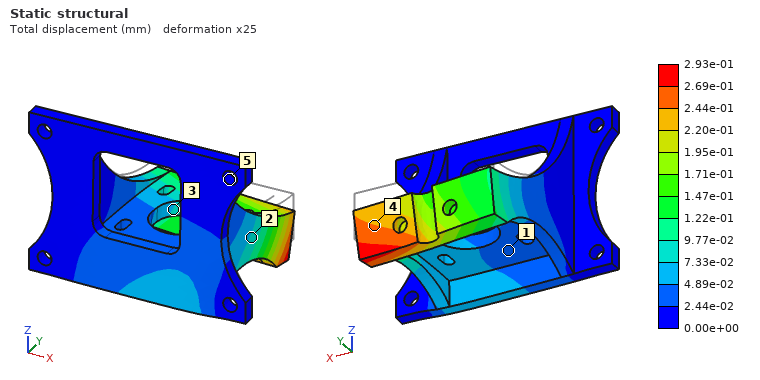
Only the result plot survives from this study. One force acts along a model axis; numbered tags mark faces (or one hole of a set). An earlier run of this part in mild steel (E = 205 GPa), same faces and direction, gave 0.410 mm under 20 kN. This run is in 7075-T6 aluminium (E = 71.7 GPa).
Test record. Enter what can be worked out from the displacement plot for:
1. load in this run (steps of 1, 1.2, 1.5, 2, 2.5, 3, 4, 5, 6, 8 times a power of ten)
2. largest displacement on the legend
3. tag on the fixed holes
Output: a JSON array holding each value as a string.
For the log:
["5 kN", "2.93e-01 mm", "5"]
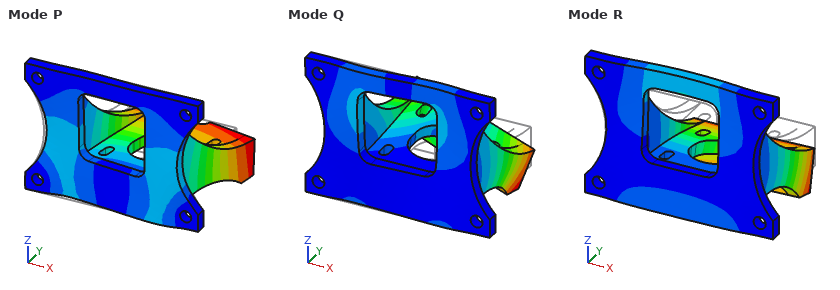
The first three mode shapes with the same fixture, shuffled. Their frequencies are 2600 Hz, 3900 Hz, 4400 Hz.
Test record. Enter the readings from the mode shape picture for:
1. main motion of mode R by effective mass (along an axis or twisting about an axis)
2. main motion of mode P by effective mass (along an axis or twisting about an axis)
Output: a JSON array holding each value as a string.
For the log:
["along Z", "along X"]
